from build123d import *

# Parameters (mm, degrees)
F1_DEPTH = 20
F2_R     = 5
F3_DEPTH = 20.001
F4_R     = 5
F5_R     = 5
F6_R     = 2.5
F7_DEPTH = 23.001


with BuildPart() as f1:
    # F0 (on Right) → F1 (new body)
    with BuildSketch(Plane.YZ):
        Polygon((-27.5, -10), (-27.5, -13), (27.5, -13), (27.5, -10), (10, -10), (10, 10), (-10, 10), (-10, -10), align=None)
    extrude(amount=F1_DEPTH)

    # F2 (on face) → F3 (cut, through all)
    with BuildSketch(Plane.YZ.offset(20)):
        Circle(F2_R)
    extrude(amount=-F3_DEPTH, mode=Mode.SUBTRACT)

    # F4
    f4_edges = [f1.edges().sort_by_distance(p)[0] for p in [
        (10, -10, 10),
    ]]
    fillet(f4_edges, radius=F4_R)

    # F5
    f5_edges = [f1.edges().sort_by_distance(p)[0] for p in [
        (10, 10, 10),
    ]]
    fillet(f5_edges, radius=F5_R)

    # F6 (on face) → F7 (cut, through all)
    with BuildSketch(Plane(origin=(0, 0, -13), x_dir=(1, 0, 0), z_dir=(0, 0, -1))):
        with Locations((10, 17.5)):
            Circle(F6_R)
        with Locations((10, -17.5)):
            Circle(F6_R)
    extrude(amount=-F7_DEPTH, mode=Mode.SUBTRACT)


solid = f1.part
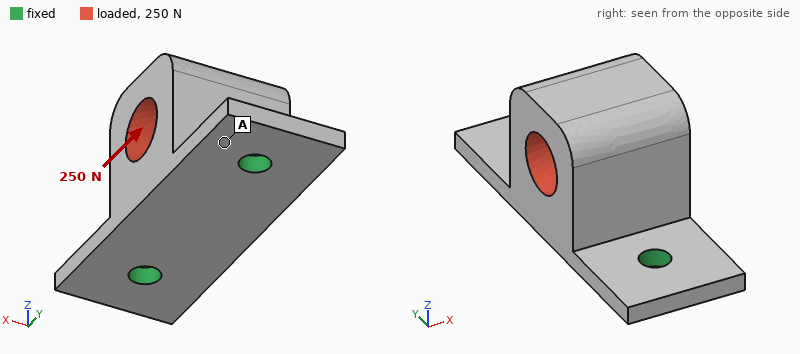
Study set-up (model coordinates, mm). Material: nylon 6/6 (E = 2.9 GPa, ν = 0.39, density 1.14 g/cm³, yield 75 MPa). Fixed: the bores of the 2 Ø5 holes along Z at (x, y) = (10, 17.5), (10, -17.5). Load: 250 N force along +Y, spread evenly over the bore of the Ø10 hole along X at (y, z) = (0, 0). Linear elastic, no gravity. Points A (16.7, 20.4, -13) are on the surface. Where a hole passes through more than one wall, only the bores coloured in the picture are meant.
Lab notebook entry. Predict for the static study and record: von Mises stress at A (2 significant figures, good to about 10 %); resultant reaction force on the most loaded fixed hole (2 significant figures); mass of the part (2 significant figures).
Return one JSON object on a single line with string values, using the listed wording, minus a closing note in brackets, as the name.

{"von Mises stress at A": "2.4 MPa", "resultant reaction force on the most loaded fixed hole": "170 N", "mass of the part": "11 g"}
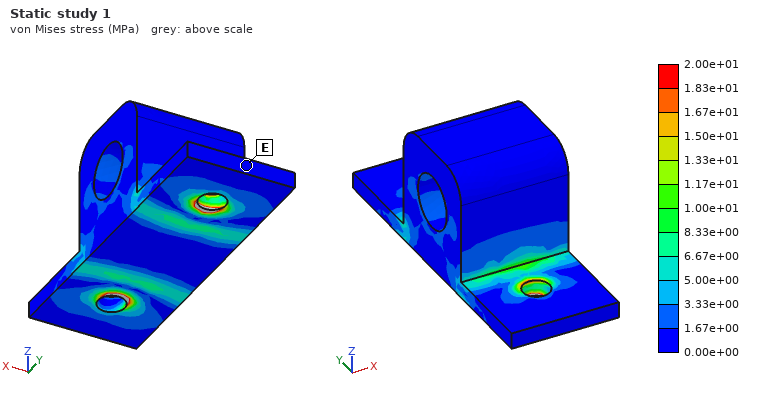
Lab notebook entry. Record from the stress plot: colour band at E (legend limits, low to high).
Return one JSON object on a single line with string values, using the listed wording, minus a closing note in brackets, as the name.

{"colour band at E": "0.00e+00 to 1.67e+00 MPa"}
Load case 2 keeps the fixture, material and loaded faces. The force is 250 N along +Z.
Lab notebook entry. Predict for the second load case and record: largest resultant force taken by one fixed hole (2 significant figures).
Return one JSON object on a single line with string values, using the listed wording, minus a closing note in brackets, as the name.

{"largest resultant force taken by one fixed hole": "140 N"}
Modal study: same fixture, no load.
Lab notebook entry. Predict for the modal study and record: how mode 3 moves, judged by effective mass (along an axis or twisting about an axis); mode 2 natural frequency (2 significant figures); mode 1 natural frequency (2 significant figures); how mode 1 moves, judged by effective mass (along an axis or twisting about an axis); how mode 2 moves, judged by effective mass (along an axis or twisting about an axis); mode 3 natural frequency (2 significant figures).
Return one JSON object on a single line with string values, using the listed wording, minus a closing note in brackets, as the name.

{"how mode 3 moves, judged by effective mass": "along Z", "mode 2 natural frequency": "3000 Hz", "mode 1 natural frequency": "1200 Hz", "how mode 1 moves, judged by effective mass": "along X", "how mode 2 moves, judged by effective mass": "along Y", "mode 3 natural frequency": "3200 Hz"}
